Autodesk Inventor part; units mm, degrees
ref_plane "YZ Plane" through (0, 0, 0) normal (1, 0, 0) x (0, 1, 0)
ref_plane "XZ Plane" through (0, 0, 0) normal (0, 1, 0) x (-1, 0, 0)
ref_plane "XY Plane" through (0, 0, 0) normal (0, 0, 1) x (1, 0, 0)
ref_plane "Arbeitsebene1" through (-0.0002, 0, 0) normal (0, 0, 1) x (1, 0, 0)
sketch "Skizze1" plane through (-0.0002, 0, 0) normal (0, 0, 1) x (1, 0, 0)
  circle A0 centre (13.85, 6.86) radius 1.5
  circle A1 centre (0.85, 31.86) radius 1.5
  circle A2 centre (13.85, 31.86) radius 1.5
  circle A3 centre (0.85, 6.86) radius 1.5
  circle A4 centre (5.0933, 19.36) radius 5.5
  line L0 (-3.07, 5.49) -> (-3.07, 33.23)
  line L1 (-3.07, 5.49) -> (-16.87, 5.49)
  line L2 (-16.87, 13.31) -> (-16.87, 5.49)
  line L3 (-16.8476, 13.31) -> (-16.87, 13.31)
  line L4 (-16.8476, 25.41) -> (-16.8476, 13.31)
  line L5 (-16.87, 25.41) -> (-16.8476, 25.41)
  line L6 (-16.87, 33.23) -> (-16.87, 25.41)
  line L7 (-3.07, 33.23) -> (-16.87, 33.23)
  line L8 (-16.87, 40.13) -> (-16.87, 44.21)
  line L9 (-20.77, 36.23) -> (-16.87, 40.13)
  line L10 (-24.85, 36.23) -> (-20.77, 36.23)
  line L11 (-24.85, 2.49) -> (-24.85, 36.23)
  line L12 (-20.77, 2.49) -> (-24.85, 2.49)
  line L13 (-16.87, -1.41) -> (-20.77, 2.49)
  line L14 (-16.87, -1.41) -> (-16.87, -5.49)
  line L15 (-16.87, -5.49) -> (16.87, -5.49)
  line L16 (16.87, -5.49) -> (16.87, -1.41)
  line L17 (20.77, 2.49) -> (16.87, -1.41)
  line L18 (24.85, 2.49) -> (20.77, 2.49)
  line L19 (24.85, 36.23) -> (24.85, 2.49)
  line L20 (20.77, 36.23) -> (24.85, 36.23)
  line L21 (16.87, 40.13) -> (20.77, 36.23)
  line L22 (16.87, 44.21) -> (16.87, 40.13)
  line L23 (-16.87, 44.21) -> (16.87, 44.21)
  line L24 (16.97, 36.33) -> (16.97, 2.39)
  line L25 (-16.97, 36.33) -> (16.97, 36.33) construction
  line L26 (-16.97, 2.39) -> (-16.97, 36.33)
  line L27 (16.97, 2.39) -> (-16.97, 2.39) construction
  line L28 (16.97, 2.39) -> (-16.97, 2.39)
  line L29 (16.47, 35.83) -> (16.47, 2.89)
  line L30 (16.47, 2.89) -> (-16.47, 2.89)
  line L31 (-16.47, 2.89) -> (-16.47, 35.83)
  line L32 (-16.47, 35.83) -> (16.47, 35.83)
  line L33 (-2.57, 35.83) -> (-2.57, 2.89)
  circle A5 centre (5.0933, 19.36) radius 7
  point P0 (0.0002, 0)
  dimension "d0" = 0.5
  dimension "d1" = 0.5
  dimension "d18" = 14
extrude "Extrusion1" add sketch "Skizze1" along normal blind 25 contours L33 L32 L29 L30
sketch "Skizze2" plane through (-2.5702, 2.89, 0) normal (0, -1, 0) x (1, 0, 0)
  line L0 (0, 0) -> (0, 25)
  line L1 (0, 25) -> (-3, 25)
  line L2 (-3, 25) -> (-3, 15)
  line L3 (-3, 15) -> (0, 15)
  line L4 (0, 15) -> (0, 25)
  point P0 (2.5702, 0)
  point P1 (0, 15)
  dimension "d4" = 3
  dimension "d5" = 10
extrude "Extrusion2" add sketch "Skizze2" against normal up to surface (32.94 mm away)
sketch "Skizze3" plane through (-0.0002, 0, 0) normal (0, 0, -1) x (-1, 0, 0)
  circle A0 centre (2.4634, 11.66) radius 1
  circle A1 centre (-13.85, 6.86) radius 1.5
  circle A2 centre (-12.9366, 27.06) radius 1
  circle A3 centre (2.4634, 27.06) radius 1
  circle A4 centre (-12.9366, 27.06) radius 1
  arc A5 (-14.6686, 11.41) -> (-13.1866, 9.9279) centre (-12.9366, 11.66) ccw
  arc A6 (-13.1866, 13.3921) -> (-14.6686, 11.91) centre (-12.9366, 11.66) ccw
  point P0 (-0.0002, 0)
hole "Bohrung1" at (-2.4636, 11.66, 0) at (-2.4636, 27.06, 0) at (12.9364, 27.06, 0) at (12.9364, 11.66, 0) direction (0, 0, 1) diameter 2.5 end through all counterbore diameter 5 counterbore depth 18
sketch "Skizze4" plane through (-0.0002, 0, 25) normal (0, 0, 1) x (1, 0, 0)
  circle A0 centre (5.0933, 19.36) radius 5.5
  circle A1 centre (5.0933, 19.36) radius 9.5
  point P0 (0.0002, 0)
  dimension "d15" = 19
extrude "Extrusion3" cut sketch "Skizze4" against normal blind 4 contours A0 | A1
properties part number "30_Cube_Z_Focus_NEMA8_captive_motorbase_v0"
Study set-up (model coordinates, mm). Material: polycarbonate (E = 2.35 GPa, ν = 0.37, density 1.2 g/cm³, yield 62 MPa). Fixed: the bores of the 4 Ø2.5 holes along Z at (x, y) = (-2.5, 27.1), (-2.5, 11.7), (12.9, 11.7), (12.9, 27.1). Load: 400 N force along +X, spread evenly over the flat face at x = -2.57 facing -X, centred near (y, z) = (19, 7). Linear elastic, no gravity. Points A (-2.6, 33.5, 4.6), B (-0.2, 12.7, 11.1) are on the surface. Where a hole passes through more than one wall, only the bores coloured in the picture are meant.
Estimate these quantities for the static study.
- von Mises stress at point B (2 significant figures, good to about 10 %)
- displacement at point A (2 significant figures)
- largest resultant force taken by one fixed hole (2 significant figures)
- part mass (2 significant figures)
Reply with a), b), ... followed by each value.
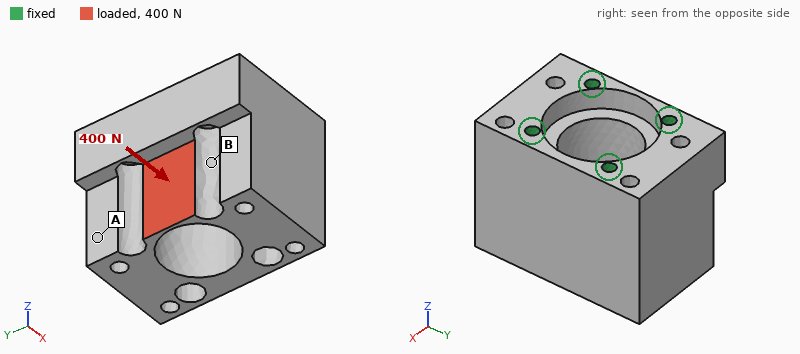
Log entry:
a) 7.2 MPa
b) 0.077 mm
c) 210 N
d) 12 g
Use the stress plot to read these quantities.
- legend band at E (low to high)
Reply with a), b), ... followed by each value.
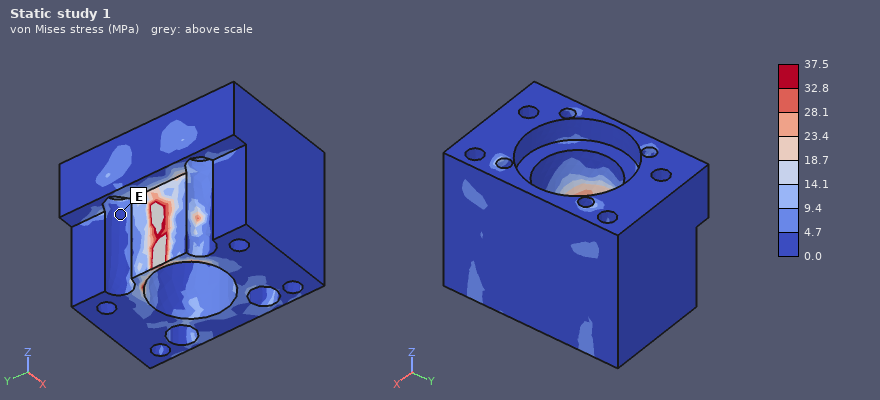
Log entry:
a) 0.0 to 4.7 MPa
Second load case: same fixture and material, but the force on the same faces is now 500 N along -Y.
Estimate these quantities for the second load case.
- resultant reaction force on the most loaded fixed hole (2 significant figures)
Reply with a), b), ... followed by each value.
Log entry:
a) 240 N
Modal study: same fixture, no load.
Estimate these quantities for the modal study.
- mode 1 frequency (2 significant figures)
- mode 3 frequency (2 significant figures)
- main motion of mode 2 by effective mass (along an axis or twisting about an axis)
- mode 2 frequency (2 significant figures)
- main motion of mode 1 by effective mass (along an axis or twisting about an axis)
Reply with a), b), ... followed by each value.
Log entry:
a) 4400 Hz
b) 6200 Hz
c) along X
d) 5200 Hz
e) along Y
